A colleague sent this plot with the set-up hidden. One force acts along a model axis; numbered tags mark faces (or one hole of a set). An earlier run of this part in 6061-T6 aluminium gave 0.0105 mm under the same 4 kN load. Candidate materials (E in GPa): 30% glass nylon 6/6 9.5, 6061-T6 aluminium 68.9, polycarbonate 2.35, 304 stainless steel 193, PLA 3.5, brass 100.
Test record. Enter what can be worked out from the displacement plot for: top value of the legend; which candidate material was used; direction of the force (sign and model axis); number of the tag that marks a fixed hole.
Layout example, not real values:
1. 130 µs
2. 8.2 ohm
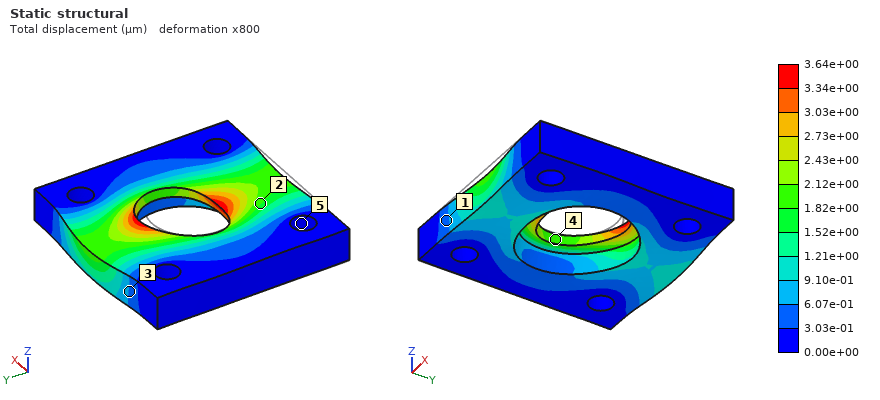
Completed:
1. 3.64e+00 µm
2. 304 stainless steel
3. +Y
4. 5
